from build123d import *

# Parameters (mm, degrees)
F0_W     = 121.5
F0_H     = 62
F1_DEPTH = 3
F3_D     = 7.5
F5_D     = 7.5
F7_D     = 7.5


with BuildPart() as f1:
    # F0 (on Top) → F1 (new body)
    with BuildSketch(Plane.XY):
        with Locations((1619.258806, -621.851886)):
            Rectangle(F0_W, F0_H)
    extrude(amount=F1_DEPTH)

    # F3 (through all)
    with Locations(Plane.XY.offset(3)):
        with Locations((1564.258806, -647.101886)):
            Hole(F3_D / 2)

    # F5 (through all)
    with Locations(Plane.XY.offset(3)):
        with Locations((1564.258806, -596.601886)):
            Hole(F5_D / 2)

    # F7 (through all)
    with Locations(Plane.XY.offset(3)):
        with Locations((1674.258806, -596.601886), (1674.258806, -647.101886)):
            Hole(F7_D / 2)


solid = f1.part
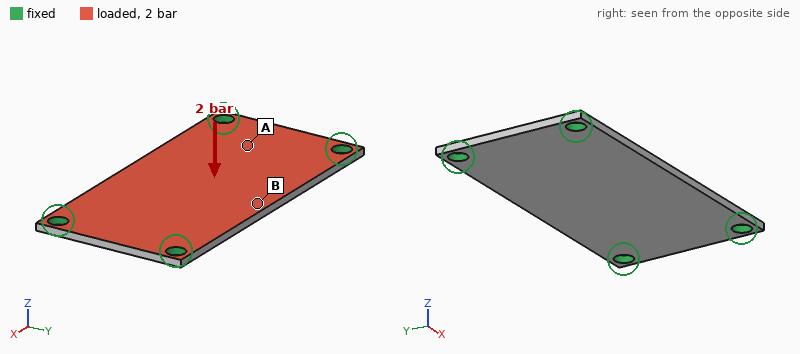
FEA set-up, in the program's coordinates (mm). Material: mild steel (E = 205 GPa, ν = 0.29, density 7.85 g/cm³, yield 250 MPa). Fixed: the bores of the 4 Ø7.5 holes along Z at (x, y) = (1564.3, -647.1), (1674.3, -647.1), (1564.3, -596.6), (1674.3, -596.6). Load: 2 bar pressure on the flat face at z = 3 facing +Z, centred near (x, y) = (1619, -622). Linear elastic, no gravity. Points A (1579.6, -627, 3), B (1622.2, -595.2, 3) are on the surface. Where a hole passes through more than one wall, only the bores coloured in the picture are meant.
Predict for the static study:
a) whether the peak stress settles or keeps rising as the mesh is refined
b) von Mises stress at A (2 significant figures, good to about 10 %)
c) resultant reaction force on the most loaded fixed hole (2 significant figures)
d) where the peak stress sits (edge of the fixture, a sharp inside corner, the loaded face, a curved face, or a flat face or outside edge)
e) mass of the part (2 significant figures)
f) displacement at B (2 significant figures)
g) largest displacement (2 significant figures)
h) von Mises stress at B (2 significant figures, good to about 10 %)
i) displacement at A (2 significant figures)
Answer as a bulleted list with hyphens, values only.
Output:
- keeps rising
- 33 MPa
- 370 N
- edge of the fixture
- 170 g
- 0.17 mm
- 0.17 mm
- 70 MPa
- 0.052 mm
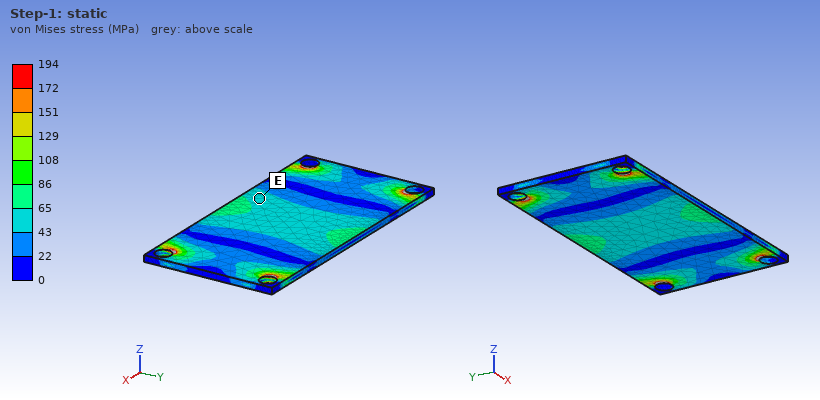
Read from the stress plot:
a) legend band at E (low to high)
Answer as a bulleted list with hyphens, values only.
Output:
- 43 to 65 MPa
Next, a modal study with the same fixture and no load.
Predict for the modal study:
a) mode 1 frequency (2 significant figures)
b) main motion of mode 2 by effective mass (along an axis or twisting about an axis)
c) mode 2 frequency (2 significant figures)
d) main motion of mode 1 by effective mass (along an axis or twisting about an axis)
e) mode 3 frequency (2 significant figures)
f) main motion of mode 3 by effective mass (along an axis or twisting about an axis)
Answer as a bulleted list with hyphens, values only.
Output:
- 1300 Hz
- twisting about X
- 2100 Hz
- along Z
- 3500 Hz
- twisting about Y
